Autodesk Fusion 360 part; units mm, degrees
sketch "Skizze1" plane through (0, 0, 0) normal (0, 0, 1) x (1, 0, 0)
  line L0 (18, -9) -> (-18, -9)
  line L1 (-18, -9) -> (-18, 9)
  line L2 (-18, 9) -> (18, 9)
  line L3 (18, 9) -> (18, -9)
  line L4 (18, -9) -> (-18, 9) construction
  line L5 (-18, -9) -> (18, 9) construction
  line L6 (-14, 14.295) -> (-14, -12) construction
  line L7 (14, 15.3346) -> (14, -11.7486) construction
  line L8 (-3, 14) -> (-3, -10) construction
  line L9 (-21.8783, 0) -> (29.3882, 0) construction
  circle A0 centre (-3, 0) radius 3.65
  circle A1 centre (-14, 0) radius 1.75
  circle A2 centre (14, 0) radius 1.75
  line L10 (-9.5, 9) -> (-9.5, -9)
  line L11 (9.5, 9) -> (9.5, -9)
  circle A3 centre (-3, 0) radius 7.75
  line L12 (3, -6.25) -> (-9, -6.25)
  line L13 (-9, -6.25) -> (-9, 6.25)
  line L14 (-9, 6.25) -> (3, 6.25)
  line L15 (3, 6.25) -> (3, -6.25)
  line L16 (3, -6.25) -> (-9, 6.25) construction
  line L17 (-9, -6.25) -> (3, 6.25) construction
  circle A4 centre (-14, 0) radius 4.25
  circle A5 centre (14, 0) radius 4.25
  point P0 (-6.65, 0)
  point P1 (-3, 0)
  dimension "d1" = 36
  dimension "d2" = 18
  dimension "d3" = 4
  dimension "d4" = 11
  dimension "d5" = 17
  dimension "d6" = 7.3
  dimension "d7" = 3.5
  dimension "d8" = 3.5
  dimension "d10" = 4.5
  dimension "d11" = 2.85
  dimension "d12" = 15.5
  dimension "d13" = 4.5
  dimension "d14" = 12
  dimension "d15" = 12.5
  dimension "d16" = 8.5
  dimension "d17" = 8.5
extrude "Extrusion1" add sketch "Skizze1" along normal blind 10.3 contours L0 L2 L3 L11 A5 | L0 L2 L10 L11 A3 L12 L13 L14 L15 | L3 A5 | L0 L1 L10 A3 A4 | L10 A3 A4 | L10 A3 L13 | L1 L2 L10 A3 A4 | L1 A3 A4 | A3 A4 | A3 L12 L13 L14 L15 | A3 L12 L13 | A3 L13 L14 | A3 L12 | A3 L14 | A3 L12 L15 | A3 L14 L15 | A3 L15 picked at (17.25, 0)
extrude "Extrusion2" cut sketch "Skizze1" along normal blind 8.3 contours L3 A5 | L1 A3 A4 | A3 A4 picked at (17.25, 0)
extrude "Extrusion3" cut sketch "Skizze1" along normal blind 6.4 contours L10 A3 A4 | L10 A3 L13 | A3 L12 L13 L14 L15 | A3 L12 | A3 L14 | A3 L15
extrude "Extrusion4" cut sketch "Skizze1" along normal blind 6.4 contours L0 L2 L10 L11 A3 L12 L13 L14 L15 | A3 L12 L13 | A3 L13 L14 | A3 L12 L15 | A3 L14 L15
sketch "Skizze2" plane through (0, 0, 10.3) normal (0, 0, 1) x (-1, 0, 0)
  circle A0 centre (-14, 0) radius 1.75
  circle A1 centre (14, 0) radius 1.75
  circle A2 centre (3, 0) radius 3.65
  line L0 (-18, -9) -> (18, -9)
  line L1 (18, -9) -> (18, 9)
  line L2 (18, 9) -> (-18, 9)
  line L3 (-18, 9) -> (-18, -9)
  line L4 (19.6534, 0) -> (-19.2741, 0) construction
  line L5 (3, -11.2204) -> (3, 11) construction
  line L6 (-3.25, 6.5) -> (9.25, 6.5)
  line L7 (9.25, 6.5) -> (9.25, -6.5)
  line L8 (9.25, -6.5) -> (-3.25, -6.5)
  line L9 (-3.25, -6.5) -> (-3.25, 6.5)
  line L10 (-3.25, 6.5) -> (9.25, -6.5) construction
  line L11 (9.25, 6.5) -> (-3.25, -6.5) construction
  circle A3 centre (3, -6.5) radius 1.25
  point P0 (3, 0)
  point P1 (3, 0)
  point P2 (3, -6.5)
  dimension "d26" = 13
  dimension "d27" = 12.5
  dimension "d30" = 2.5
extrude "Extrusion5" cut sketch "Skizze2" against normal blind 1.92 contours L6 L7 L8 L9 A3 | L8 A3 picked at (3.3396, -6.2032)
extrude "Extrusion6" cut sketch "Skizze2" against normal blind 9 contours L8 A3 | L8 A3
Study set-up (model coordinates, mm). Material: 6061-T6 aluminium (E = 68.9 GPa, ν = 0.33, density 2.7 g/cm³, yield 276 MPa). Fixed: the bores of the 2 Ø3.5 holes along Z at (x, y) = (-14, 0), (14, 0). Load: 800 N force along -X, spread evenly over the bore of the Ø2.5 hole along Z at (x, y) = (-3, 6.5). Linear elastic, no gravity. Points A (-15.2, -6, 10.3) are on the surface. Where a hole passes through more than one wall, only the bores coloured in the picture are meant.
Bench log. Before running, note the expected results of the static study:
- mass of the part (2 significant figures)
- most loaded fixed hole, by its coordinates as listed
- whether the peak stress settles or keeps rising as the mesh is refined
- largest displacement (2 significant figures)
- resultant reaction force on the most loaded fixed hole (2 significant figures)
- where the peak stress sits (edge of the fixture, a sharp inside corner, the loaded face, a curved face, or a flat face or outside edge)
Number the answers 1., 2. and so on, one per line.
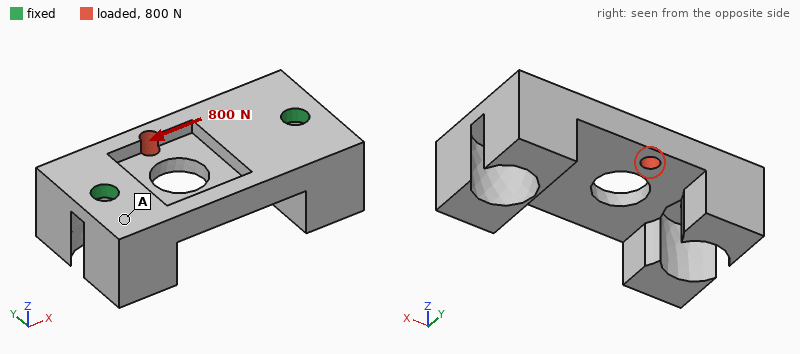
1. 8.3 g
2. (14, 0)
3. keeps rising
4. 12 µm
5. 460 N
6. edge of the fixture
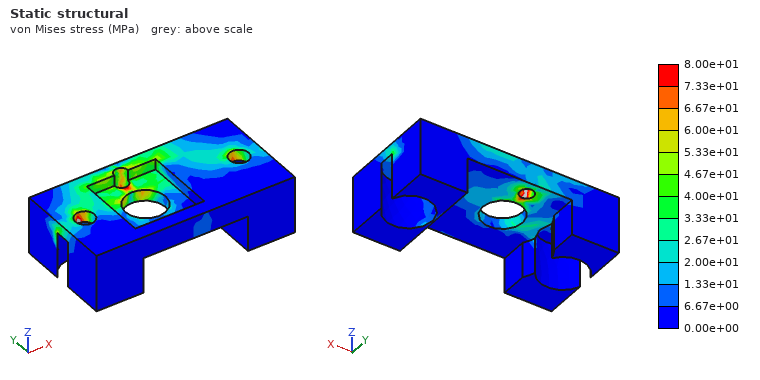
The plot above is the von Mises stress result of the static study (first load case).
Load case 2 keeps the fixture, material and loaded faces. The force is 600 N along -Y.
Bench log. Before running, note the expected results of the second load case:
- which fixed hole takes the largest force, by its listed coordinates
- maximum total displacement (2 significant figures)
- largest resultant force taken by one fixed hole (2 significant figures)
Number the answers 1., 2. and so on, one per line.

1. (-14, 0)
2. 17 µm
3. 370 N
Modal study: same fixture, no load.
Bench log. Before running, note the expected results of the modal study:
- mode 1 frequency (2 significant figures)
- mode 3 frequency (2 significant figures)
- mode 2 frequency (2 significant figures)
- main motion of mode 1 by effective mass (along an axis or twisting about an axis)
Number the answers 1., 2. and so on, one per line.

1. 8100 Hz
2. 12 kHz
3. 12 kHz
4. along Y
